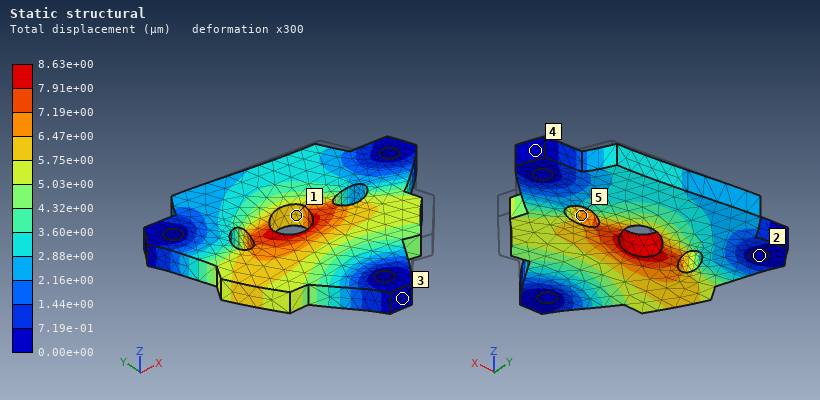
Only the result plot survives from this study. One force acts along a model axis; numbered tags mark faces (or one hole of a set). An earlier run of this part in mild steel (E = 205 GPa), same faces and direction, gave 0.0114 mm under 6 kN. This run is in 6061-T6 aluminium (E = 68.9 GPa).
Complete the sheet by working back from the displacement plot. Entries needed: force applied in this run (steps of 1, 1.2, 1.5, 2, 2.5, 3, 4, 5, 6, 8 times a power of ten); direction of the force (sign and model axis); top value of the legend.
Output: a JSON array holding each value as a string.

["1.5 kN", "-X", "8.63e+00 µm"]
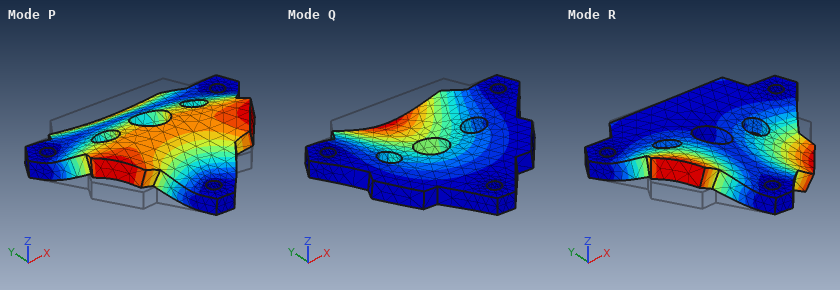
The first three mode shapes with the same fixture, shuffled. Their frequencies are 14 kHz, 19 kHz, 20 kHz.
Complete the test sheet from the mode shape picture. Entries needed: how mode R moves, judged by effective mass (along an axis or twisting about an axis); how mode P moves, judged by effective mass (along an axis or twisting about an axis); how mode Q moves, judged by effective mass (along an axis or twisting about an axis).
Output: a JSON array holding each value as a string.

["twisting about Y", "along Z", "along Z"]
